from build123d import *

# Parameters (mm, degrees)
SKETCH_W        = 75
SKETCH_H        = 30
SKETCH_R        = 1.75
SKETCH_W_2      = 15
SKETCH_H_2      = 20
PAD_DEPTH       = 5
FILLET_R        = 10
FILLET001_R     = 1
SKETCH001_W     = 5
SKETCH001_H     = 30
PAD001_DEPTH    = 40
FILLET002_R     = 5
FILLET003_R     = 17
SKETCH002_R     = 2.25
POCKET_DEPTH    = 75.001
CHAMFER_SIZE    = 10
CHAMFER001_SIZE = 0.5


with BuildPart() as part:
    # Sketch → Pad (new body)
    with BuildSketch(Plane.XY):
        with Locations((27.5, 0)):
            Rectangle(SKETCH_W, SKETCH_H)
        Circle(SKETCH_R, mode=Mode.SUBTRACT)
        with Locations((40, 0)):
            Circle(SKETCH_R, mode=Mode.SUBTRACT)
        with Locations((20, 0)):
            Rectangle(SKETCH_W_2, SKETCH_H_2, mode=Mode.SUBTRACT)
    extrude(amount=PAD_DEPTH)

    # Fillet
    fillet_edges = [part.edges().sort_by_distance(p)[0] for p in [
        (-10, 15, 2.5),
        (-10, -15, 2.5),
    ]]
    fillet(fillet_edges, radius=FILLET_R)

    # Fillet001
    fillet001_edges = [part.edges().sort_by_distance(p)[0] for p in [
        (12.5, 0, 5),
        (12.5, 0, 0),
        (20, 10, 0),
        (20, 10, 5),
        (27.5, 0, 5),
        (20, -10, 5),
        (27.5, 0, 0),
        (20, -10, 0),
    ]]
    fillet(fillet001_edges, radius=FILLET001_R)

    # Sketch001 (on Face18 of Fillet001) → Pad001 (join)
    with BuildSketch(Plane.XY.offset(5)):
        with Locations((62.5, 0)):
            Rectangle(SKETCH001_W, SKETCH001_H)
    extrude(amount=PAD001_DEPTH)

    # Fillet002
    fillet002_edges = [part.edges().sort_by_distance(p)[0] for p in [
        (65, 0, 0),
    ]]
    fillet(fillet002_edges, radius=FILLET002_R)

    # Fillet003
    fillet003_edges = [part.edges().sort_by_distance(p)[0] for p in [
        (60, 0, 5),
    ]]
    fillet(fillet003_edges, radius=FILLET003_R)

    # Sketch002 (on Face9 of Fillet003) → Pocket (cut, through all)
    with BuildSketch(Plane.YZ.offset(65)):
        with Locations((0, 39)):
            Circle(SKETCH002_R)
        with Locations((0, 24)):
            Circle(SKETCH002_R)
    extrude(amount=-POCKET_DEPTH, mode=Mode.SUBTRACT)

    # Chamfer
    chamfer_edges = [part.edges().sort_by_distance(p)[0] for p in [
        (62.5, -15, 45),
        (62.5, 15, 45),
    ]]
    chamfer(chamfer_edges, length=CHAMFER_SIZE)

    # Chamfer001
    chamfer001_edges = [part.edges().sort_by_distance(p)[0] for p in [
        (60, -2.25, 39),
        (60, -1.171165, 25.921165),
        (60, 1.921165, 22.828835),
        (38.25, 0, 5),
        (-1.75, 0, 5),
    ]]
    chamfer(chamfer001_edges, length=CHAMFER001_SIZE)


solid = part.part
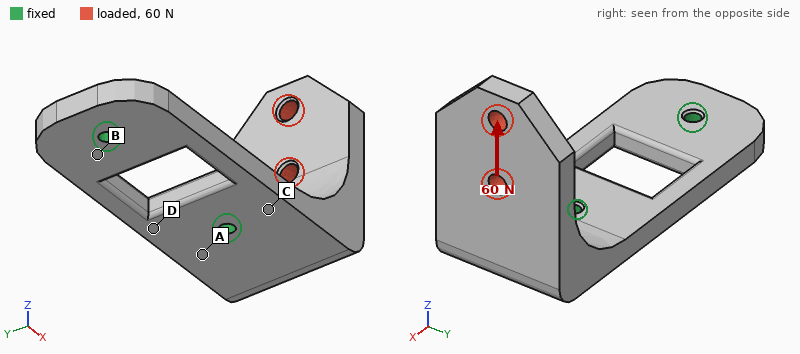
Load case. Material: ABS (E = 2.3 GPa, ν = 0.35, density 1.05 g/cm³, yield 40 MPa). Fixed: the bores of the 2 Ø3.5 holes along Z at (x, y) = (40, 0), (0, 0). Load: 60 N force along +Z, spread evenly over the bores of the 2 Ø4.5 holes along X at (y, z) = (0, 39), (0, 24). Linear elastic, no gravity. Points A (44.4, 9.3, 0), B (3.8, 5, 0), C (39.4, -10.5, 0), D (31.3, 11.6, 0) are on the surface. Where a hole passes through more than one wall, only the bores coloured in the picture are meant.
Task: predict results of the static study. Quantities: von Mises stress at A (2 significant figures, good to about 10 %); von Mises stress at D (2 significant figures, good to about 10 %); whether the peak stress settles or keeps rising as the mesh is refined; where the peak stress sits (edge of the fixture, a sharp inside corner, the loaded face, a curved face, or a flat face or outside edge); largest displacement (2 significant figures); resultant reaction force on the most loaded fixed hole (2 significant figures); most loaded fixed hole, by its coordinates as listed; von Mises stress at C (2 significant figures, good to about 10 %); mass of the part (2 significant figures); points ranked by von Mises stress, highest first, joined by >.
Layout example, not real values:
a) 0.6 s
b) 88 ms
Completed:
a) 6.1 MPa
b) 2.6 MPa
c) keeps rising
d) edge of the fixture
e) 0.93 mm
f) 69 N
g) (40, 0)
h) 4.8 MPa
i) 17 g
j) A > C > D > B
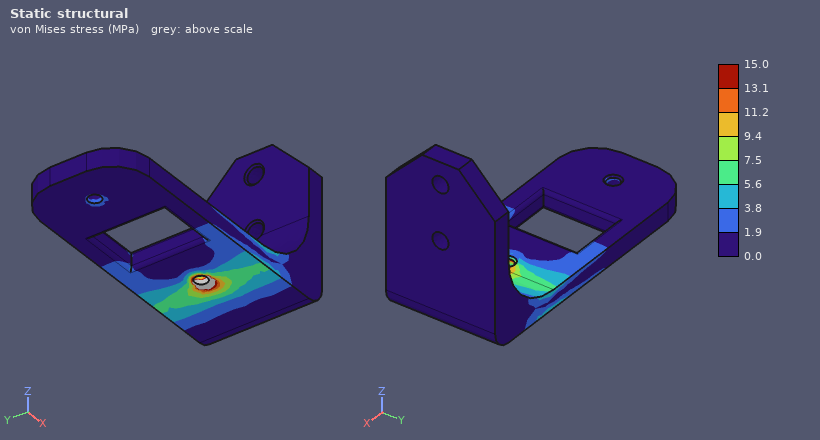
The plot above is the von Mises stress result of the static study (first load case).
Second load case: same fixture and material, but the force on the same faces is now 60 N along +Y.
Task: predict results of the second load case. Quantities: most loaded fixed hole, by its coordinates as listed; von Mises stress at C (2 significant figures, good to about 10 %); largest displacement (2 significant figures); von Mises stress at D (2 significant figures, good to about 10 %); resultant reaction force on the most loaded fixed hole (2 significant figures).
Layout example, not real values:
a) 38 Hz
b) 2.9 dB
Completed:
a) (40, 0)
b) 5.1 MPa
c) 1.0 mm
d) 2.6 MPa
e) 78 N
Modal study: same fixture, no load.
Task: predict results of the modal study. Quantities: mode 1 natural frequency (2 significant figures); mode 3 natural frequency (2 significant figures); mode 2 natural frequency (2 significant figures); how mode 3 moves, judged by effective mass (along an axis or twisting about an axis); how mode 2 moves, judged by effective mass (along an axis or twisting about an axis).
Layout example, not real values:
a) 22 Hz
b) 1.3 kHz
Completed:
a) 490 Hz
b) 1700 Hz
c) 690 Hz
d) along Z
e) along Y
